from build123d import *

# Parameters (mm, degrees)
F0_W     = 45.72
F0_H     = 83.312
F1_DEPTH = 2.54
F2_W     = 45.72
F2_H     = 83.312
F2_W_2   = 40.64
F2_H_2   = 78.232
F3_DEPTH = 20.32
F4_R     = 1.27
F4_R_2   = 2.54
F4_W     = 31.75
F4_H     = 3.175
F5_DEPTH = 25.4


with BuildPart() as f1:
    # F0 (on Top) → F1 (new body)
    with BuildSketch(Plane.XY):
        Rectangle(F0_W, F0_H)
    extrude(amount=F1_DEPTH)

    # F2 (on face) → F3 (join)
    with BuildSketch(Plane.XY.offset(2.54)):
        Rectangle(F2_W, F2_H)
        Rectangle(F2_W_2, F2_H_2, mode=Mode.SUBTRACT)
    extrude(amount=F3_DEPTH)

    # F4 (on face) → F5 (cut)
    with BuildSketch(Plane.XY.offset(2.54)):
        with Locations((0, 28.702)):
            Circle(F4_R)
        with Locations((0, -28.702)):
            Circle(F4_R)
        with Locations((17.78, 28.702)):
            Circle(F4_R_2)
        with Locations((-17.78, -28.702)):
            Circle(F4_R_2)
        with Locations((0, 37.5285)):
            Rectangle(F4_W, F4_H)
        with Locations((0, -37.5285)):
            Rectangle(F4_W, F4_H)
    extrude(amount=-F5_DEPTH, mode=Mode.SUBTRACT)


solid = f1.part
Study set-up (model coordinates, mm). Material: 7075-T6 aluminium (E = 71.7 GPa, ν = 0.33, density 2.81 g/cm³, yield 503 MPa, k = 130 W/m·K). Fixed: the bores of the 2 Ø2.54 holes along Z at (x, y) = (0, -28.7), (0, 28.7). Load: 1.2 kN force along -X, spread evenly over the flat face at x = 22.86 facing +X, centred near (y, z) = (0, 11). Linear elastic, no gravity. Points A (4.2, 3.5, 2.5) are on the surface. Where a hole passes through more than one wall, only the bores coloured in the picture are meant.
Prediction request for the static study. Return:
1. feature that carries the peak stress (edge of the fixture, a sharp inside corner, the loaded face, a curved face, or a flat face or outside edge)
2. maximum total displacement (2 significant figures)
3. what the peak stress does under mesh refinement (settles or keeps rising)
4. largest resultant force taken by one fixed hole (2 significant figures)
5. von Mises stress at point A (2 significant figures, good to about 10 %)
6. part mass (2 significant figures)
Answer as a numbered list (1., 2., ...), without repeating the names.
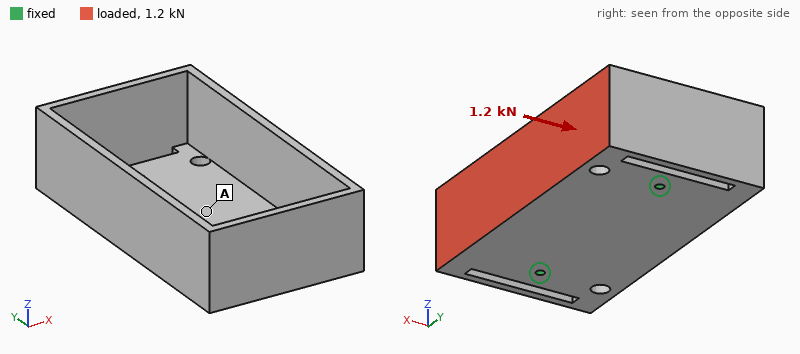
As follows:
1. edge of the fixture
2. 0.67 mm
3. keeps rising
4. 600 N
5. 34 MPa
6. 61 g
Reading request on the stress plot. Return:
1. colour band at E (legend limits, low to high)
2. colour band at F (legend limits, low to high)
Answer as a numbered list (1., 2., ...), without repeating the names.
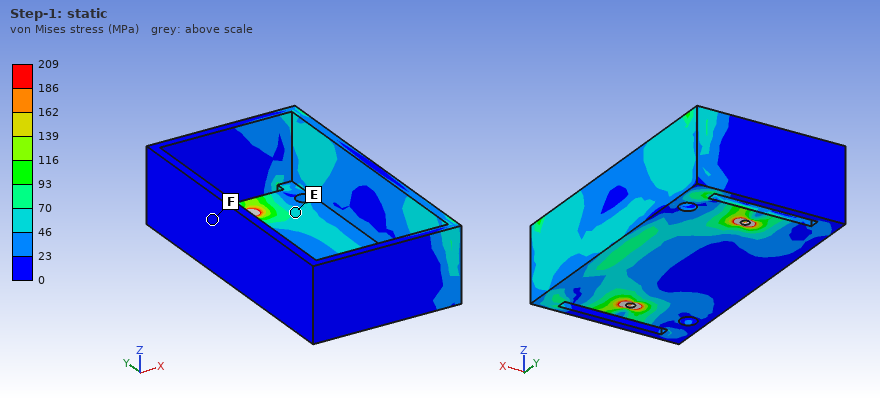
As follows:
1. 46 to 70 MPa
2. 0 to 23 MPa
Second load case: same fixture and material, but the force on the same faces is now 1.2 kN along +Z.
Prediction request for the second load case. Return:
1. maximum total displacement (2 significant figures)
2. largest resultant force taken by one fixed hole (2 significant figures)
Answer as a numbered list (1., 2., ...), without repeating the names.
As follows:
1. 1.1 mm
2. 600 N
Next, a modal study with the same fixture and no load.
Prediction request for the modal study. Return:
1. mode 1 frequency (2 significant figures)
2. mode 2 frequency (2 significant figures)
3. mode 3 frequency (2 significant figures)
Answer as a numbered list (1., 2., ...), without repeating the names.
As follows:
1. 1000 Hz
2. 1800 Hz
3. 2000 Hz
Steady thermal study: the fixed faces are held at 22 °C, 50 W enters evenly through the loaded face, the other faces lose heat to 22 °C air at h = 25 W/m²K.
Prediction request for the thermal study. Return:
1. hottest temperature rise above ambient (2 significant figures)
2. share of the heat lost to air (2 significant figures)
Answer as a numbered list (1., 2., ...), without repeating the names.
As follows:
1. 65 K
2. 26 %
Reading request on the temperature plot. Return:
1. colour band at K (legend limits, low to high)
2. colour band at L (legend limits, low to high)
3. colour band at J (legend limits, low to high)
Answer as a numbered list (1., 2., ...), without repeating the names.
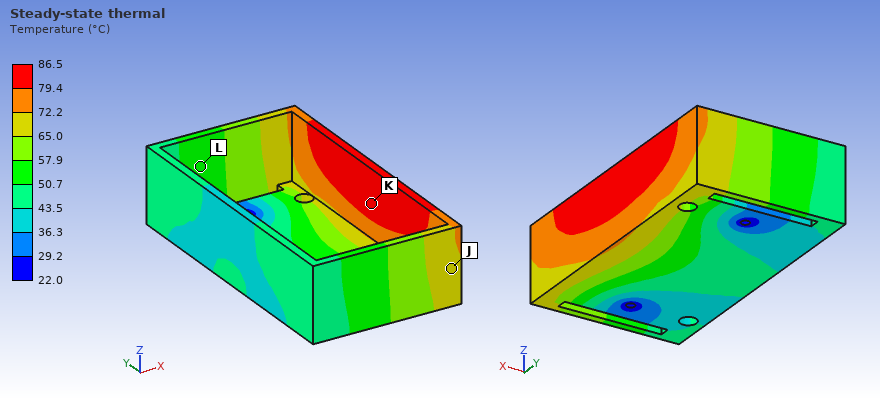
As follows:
1. 79.4 to 86.5 °C
2. 50.7 to 57.9 °C
3. 65.0 to 72.2 °C
